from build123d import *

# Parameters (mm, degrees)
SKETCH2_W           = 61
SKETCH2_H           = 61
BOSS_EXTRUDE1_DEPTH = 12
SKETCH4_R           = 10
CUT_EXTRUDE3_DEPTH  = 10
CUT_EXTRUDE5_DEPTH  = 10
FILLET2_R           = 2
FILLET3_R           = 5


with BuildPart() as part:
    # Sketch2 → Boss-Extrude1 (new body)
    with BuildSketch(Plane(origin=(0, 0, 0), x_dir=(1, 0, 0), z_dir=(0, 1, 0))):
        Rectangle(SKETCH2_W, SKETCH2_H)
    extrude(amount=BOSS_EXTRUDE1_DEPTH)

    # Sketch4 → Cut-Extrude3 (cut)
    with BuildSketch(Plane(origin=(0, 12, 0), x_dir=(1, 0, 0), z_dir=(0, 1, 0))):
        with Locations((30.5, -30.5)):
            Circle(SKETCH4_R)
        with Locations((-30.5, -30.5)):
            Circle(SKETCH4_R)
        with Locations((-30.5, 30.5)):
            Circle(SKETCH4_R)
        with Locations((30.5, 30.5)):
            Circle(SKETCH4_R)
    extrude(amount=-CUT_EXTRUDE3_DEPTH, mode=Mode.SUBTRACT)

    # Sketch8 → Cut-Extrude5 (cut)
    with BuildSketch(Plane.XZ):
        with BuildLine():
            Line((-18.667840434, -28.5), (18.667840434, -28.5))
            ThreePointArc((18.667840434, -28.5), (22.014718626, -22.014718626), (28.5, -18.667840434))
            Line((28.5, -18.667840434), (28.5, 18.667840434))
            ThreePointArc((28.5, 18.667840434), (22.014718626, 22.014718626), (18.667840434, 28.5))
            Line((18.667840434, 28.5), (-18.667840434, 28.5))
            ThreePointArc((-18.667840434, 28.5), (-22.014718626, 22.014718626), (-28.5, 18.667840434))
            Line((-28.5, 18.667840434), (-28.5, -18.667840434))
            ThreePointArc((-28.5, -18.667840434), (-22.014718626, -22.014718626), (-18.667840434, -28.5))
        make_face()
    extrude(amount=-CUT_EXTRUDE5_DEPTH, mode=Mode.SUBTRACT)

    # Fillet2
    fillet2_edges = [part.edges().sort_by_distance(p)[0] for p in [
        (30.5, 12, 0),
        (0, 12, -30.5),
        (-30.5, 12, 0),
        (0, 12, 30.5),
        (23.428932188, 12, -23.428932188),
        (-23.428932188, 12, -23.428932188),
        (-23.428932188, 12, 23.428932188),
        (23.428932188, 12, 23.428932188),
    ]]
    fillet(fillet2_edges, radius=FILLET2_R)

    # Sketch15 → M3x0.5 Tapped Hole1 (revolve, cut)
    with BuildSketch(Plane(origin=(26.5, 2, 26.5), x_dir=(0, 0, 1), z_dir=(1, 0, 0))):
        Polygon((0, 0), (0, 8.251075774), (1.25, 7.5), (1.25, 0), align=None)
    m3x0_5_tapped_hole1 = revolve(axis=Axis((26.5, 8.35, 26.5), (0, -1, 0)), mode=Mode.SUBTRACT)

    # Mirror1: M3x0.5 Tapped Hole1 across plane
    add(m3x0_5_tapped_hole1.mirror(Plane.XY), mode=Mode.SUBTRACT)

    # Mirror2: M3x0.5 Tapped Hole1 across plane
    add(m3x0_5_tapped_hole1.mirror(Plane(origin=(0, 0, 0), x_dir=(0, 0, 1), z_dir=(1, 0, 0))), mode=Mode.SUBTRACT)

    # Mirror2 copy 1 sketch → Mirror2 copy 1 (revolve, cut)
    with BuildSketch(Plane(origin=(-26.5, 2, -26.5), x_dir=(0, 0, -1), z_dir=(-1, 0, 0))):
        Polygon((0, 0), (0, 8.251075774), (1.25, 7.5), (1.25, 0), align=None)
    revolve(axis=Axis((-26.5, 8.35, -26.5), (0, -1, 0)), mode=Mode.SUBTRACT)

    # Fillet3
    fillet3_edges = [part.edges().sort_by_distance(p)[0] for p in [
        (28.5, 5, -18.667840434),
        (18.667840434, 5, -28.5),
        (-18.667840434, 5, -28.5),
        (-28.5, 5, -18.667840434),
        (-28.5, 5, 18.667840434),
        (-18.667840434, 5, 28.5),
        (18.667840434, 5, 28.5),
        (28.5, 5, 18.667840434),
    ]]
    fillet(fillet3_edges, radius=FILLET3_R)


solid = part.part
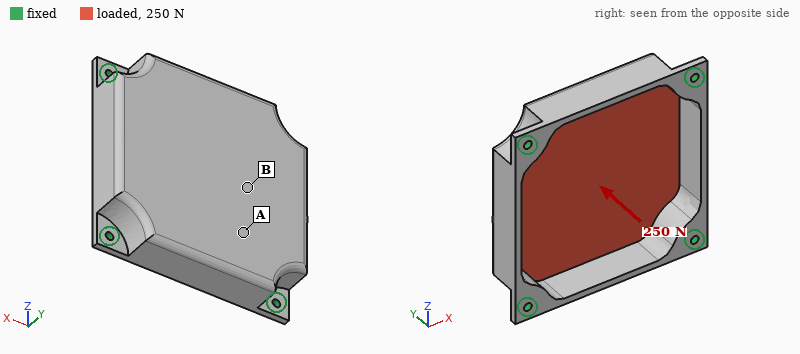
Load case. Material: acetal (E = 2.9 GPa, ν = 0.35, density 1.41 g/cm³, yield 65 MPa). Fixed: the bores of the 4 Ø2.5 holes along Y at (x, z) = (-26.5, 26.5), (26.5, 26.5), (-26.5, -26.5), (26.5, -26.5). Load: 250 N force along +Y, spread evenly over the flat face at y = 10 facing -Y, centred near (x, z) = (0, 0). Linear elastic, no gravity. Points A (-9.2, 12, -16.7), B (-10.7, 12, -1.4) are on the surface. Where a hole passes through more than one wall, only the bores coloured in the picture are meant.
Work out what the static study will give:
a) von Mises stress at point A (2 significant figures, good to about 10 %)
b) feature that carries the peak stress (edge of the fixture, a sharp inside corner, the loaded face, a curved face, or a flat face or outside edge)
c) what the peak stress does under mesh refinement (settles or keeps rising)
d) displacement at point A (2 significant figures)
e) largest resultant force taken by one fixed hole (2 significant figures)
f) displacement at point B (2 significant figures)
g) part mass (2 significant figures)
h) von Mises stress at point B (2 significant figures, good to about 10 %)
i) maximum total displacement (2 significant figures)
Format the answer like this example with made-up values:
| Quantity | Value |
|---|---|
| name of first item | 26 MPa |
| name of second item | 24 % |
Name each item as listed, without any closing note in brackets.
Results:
| Quantity | Value |
|---|---|
| von Mises stress at point A | 6.8 MPa |
| feature that carries the peak stress | edge of the fixture |
| what the peak stress does under mesh refinement | keeps rising |
| displacement at point A | 0.45 mm |
| largest resultant force taken by one fixed hole | 79 N |
| displacement at point B | 0.74 mm |
| part mass | 17 g |
| von Mises stress at point B | 11 MPa |
| maximum total displacement | 0.90 mm |
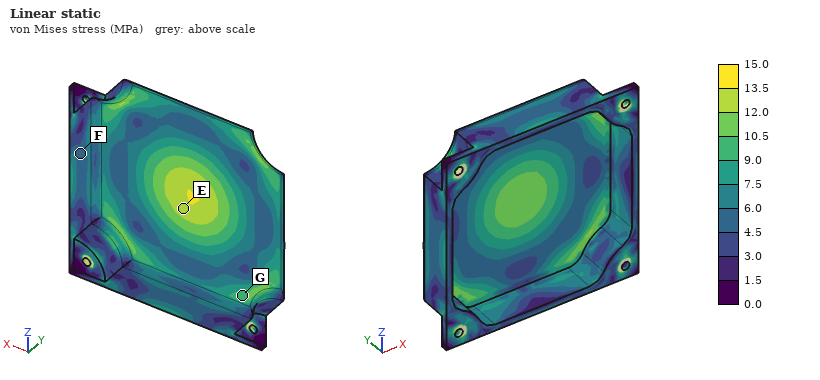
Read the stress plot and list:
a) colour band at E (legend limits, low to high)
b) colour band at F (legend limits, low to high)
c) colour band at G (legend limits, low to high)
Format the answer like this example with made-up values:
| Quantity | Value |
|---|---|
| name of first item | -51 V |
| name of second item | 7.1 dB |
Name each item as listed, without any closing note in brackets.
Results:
| Quantity | Value |
|---|---|
| colour band at E | 12.0 to 13.5 MPa |
| colour band at F | 4.5 to 6.0 MPa |
| colour band at G | 9.0 to 10.5 MPa |
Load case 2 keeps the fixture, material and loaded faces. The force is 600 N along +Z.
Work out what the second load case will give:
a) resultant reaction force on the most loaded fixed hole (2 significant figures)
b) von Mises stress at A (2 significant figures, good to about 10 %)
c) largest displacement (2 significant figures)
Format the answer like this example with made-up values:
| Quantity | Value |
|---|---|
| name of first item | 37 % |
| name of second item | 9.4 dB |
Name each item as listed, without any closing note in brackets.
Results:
| Quantity | Value |
|---|---|
| resultant reaction force on the most loaded fixed hole | 160 N |
| von Mises stress at A | 2.7 MPa |
| largest displacement | 0.15 mm |
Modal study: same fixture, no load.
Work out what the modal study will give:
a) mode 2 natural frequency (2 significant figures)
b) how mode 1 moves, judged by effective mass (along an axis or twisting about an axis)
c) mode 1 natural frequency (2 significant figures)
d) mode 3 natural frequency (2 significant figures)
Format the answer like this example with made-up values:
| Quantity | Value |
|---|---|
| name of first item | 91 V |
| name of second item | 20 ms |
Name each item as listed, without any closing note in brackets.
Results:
| Quantity | Value |
|---|---|
| mode 2 natural frequency | 2300 Hz |
| how mode 1 moves, judged by effective mass | along Y |
| mode 1 natural frequency | 1200 Hz |
| mode 3 natural frequency | 2300 Hz |
